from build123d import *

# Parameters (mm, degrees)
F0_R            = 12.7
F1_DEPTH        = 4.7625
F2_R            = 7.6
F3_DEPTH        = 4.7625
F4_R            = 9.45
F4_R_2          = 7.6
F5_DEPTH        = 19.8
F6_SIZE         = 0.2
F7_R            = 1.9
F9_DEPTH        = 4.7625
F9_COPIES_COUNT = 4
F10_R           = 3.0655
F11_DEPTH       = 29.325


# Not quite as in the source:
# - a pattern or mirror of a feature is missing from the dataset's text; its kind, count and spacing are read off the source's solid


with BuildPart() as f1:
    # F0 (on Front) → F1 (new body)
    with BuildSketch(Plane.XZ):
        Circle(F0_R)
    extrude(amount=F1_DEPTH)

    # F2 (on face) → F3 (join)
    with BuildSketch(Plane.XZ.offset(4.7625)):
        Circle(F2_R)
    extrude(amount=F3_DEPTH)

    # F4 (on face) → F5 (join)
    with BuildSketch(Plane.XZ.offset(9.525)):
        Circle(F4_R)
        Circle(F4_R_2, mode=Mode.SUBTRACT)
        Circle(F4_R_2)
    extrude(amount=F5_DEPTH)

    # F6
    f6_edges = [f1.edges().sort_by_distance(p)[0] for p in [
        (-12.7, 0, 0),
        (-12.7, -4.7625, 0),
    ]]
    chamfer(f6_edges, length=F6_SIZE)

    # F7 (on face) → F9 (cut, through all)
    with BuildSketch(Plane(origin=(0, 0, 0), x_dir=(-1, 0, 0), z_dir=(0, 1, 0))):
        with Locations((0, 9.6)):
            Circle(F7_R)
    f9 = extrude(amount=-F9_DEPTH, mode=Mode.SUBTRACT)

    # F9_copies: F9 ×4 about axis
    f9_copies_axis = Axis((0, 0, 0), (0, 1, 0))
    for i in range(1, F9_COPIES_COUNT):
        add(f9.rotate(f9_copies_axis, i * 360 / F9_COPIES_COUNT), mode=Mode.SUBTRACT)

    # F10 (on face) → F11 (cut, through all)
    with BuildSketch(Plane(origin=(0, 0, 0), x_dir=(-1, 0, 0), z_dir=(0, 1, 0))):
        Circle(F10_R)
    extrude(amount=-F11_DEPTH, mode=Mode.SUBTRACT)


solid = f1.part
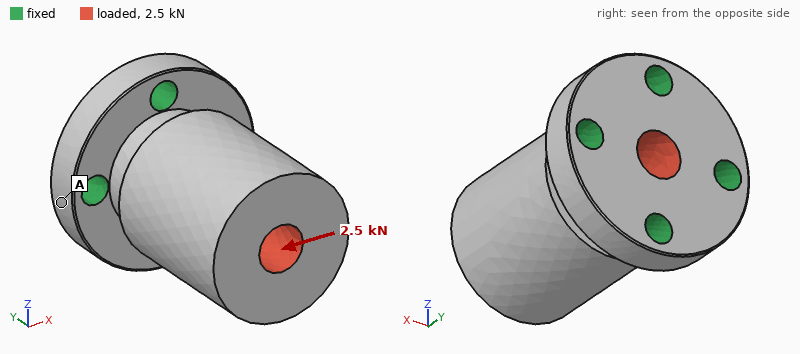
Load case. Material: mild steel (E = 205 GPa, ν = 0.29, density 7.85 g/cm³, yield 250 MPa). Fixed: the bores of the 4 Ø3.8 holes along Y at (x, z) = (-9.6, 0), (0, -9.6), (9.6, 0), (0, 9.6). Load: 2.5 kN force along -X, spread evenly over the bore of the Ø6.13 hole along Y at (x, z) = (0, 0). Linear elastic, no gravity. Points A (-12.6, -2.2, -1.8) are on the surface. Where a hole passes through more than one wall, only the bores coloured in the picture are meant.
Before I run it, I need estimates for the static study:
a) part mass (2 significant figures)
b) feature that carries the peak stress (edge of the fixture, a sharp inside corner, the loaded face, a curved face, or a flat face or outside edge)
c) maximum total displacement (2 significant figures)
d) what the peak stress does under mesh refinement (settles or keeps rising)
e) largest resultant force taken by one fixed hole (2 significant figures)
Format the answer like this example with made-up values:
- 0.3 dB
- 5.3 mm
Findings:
- 61 g
- edge of the fixture
- 15 µm
- keeps rising
- 1.9 kN
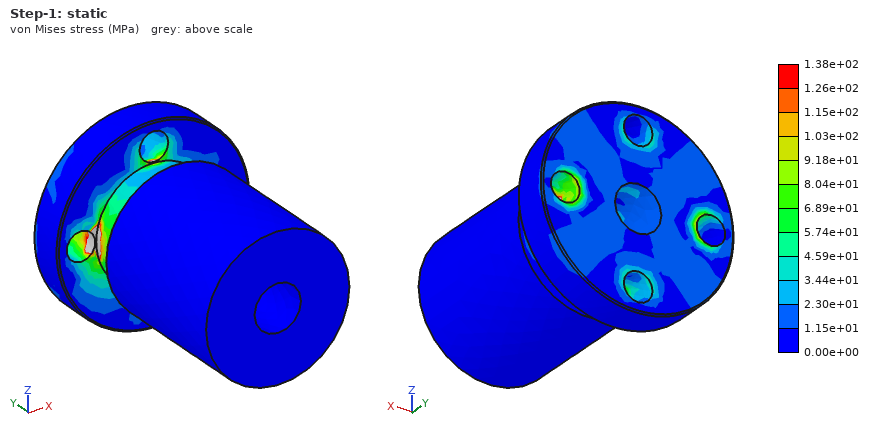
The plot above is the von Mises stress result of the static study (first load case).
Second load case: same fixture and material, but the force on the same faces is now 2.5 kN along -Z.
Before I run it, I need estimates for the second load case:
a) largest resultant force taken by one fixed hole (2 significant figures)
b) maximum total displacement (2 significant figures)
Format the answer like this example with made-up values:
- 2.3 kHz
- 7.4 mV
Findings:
- 1.9 kN
- 15 µm
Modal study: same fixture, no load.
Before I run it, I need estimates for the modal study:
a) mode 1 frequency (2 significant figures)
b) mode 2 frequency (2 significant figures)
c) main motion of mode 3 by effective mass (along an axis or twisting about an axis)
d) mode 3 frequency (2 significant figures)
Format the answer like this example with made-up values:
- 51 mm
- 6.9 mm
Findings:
- 10 kHz
- 10 kHz
- twisting about Y
- 23 kHz
